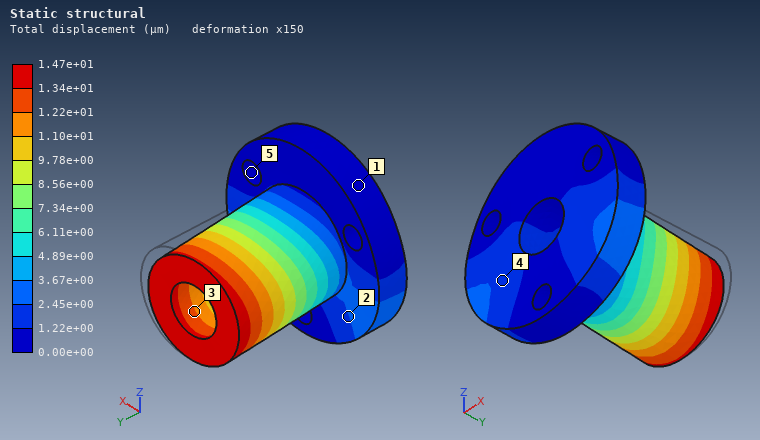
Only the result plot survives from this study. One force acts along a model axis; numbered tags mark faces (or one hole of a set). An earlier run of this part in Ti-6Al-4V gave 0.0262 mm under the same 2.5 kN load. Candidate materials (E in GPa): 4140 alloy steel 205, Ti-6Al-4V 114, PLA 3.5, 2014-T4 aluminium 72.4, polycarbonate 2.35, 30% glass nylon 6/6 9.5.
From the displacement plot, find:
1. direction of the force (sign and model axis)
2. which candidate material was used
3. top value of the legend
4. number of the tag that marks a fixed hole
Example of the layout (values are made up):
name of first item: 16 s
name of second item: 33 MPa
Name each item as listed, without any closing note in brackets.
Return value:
direction of the force: -X
which candidate material was used: 4140 alloy steel
top value of the legend: 1.47e+01 µm
number of the tag that marks a fixed hole: 5
